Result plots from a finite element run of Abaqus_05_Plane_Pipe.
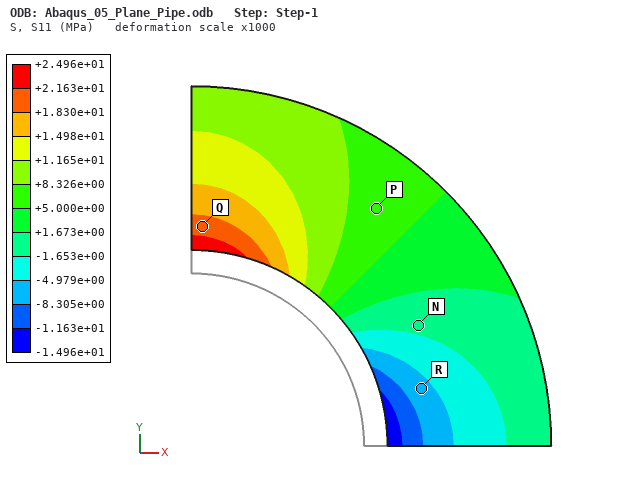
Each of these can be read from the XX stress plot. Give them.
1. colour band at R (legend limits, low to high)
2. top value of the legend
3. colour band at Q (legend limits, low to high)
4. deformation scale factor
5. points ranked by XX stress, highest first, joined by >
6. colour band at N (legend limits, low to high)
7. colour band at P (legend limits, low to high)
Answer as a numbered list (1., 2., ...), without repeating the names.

1. -8.305e+00 to -4.979e+00 MPa
2. +2.496e+01 MPa
3. +1.830e+01 to +2.163e+01 MPa
4. 1000
5. Q > P > N > R
6. -1.653e+00 to +1.673e+00 MPa
7. +5.000e+00 to +8.326e+00 MPa
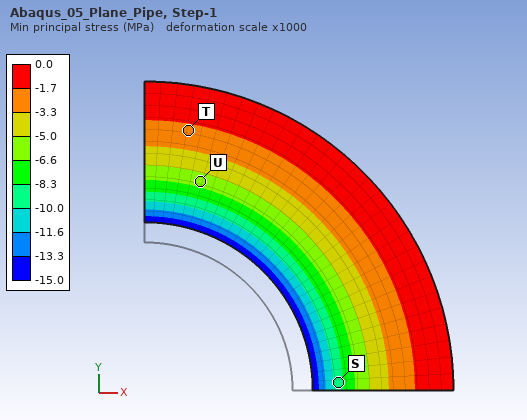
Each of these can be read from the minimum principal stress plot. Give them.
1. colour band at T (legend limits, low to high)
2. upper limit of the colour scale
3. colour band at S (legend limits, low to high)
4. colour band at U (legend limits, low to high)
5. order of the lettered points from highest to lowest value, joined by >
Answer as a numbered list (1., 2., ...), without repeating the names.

1. -3.3 to -1.7 MPa
2. 0.0 MPa
3. -10.0 to -8.3 MPa
4. -6.6 to -5.0 MPa
5. T > U > S
